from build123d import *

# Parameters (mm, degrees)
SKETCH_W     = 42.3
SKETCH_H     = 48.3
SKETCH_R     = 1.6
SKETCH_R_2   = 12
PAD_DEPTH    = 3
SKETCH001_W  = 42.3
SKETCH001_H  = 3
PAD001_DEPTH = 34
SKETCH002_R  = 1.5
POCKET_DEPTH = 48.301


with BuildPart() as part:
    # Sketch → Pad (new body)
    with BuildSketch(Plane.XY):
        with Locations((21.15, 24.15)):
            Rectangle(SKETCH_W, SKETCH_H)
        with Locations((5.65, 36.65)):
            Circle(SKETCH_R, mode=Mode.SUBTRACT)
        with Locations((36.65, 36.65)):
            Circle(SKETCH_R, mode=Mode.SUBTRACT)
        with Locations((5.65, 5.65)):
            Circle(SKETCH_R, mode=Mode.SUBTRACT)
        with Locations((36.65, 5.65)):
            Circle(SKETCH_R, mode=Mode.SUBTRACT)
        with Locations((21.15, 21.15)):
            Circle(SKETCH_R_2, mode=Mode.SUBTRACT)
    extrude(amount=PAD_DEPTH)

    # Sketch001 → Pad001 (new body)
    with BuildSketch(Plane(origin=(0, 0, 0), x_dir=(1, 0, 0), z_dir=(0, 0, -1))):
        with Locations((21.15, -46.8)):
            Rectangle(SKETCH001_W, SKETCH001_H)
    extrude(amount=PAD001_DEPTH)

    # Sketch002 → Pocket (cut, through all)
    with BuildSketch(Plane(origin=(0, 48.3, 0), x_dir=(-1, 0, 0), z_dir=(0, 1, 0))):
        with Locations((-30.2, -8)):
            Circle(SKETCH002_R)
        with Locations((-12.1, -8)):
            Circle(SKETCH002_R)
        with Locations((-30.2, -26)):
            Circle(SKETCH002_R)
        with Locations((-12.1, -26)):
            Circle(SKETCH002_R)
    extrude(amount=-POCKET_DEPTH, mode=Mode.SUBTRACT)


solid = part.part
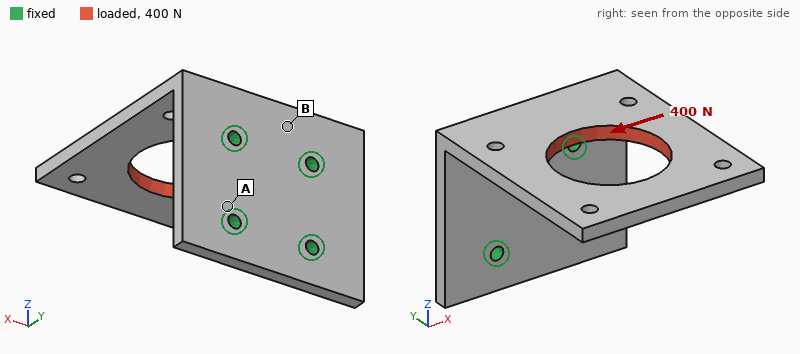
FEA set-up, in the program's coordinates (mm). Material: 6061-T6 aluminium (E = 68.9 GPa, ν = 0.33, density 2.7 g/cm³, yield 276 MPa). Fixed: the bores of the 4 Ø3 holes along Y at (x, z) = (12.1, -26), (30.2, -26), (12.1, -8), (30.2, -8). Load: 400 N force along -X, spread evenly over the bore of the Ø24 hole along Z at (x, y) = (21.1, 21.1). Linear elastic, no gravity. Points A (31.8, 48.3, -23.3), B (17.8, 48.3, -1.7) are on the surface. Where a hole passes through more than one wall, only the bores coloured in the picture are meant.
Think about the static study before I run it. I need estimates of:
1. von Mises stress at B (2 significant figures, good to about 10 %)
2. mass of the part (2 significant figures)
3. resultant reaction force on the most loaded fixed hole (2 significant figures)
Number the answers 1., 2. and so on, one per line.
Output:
1. 36 MPa
2. 24 g
3. 550 N
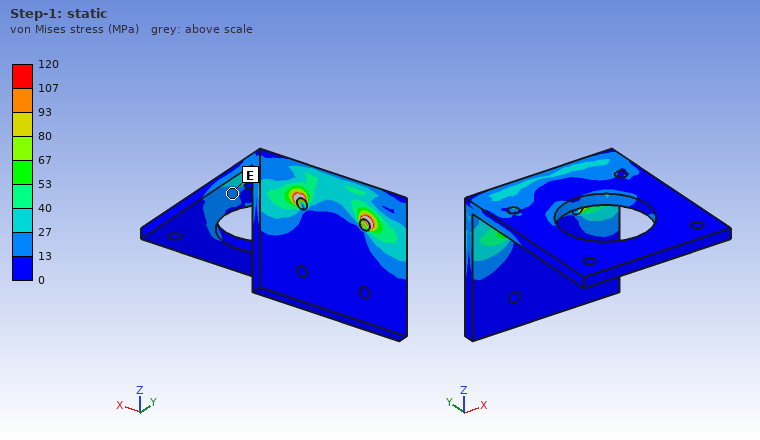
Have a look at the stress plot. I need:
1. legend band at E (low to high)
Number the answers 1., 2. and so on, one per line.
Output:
1. 13 to 27 MPa
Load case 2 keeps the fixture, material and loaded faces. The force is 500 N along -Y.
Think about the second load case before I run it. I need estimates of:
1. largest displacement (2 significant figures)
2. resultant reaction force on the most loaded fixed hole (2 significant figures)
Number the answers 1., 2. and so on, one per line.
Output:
1. 0.18 mm
2. 290 N
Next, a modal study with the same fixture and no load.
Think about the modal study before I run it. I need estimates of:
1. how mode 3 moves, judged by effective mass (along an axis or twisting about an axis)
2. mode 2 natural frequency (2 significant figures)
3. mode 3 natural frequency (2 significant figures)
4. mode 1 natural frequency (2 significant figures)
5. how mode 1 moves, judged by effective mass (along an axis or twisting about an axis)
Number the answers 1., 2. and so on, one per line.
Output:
1. along X
2. 2200 Hz
3. 3000 Hz
4. 870 Hz
5. along Z
